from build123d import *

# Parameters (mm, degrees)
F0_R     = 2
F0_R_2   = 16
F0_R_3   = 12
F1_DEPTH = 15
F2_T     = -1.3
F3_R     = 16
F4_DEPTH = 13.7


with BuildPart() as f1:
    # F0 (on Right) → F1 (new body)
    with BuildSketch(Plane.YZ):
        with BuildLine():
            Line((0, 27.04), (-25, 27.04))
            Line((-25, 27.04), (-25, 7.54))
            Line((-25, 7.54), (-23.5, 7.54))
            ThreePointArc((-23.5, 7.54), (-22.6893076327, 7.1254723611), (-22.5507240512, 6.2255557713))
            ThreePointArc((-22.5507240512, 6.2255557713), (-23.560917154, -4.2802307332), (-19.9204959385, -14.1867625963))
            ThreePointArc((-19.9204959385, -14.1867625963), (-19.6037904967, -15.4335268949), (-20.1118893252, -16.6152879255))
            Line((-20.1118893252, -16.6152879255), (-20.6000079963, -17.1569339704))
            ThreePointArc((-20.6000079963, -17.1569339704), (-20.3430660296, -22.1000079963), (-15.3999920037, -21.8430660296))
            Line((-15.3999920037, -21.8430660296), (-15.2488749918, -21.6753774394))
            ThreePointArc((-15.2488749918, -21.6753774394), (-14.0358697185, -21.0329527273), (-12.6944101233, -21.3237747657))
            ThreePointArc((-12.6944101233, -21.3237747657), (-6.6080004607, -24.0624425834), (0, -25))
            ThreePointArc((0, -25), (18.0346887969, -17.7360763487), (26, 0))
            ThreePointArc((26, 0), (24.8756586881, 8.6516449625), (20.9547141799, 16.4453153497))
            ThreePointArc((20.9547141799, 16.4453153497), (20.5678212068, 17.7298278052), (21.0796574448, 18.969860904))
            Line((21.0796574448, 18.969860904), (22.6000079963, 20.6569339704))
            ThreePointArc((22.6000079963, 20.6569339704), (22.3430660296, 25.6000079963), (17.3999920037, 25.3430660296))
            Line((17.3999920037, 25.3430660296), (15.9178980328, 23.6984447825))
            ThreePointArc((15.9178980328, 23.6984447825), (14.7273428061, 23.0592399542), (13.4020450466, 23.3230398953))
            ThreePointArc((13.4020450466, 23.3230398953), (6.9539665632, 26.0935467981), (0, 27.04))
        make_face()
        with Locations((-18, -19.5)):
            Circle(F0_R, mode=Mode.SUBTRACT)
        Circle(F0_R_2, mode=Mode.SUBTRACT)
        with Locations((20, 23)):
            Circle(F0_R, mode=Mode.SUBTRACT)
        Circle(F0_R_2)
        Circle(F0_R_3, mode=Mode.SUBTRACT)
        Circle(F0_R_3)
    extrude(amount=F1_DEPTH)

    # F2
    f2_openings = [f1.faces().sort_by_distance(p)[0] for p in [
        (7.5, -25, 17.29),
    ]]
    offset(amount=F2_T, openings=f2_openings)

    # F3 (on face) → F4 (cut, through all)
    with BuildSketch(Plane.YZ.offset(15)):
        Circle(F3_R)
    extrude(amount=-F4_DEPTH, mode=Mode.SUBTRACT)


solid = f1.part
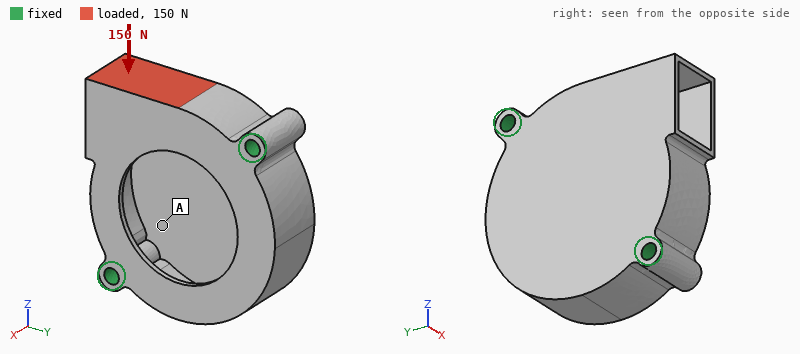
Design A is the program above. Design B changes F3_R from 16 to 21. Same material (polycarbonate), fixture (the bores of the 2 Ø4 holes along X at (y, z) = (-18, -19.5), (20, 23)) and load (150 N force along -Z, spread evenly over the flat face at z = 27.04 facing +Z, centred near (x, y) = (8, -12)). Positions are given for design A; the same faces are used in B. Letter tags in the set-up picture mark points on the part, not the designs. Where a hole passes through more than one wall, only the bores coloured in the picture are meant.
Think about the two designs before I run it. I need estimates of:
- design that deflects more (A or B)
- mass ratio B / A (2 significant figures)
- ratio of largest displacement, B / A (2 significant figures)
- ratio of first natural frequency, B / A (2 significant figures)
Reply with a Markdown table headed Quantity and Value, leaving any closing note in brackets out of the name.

| Quantity | Value |
|---|---|
| design that deflects more | B |
| mass ratio B / A | 0.90 |
| ratio of largest displacement, B / A | 1.2 |
| ratio of first natural frequency, B / A | 0.99 |
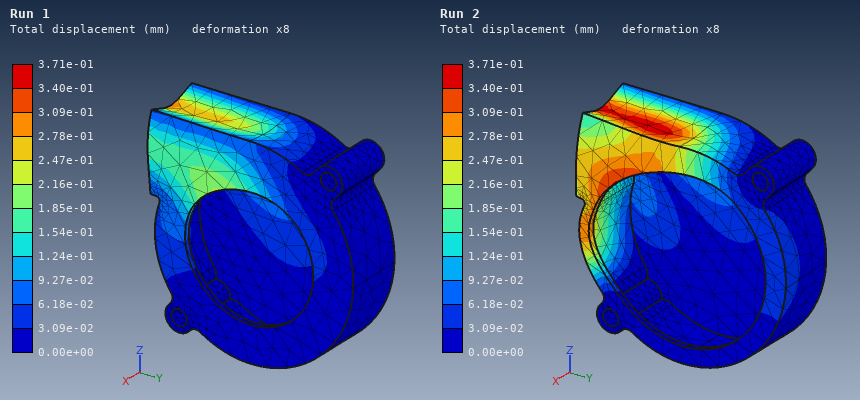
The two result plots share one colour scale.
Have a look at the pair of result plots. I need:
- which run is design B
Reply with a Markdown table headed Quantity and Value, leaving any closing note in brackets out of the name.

| Quantity | Value |
|---|---|
| which run is design B | Run 2 |
